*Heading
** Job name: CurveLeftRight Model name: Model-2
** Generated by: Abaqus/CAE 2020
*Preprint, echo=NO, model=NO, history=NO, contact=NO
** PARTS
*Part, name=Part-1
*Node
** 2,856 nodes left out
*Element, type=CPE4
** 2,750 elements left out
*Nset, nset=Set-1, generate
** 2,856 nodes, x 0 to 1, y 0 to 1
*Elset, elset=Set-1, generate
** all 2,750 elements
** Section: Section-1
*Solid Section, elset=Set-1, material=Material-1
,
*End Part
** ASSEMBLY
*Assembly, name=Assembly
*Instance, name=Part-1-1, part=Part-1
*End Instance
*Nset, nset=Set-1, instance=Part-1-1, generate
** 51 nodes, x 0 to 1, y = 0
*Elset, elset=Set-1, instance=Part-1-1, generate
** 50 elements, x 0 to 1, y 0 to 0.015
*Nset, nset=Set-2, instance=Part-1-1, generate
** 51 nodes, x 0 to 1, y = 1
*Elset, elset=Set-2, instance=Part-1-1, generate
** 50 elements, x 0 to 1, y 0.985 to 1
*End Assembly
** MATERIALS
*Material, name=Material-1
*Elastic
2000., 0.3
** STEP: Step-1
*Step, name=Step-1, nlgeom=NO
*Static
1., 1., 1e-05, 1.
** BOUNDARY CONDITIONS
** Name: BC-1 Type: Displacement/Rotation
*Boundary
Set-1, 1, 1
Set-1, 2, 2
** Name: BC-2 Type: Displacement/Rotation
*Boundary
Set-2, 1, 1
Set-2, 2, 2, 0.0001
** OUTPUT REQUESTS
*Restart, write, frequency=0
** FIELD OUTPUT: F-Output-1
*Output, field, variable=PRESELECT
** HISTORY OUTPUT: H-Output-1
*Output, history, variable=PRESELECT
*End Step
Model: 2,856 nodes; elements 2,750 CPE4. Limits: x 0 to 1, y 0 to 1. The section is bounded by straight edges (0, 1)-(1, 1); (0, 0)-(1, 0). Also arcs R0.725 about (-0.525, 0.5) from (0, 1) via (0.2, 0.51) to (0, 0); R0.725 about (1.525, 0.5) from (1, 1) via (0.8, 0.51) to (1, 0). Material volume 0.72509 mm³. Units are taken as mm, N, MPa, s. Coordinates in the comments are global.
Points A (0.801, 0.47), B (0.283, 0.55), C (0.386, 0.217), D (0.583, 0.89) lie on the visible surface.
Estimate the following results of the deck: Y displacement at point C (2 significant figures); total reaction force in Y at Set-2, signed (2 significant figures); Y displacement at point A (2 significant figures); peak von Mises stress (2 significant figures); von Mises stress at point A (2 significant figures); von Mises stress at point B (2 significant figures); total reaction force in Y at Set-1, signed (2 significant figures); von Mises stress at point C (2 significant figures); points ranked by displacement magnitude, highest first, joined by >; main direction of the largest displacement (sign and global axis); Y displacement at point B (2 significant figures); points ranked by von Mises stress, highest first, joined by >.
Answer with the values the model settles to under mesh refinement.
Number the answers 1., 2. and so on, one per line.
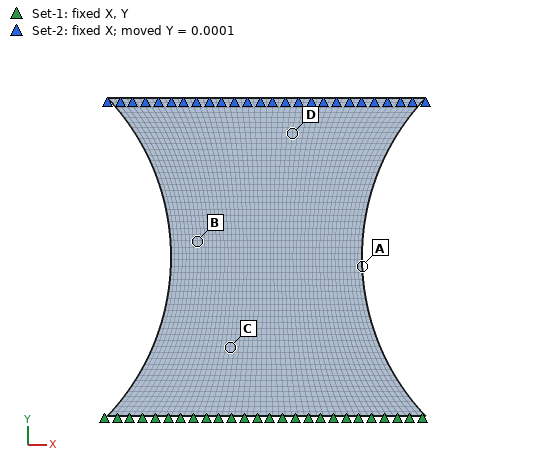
1. 2.0e-05 mm
2. 0.16 N
3. 4.6e-05 mm
4. 0.29 MPa
5. 0.29 MPa
6. 0.22 MPa
7. -0.16 N
8. 0.19 MPa
9. D > B > A > C
10. +Y
11. 5.6e-05 mm
12. A > B > C > D
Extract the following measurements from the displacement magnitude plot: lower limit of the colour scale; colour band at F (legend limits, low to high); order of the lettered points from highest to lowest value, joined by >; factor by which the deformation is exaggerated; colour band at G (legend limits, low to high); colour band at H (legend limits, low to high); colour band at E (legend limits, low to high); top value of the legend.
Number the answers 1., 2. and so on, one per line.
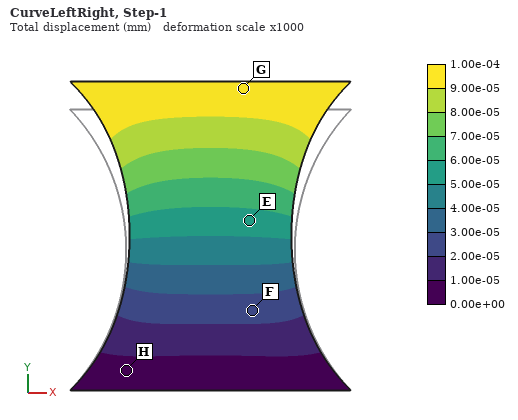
1. 0.00e+00 mm
2. 2.00e-05 to 3.00e-05 mm
3. G > E > F > H
4. 1000
5. 9.00e-05 to 1.00e-04 mm
6. 0.00e+00 to 1.00e-05 mm
7. 5.00e-05 to 6.00e-05 mm
8. 1.00e-04 mm
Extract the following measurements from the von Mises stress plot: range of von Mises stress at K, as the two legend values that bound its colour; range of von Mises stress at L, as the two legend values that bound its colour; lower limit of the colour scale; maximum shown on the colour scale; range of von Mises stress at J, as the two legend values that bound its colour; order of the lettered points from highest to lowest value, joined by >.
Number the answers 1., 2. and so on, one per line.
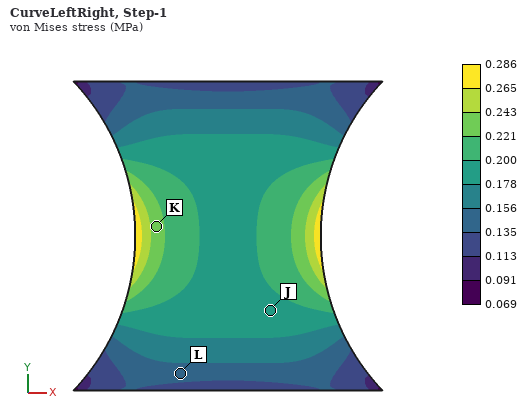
1. 0.221 to 0.243 MPa
2. 0.135 to 0.156 MPa
3. 0.069 MPa
4. 0.286 MPa
5. 0.178 to 0.200 MPa
6. K > J > L
